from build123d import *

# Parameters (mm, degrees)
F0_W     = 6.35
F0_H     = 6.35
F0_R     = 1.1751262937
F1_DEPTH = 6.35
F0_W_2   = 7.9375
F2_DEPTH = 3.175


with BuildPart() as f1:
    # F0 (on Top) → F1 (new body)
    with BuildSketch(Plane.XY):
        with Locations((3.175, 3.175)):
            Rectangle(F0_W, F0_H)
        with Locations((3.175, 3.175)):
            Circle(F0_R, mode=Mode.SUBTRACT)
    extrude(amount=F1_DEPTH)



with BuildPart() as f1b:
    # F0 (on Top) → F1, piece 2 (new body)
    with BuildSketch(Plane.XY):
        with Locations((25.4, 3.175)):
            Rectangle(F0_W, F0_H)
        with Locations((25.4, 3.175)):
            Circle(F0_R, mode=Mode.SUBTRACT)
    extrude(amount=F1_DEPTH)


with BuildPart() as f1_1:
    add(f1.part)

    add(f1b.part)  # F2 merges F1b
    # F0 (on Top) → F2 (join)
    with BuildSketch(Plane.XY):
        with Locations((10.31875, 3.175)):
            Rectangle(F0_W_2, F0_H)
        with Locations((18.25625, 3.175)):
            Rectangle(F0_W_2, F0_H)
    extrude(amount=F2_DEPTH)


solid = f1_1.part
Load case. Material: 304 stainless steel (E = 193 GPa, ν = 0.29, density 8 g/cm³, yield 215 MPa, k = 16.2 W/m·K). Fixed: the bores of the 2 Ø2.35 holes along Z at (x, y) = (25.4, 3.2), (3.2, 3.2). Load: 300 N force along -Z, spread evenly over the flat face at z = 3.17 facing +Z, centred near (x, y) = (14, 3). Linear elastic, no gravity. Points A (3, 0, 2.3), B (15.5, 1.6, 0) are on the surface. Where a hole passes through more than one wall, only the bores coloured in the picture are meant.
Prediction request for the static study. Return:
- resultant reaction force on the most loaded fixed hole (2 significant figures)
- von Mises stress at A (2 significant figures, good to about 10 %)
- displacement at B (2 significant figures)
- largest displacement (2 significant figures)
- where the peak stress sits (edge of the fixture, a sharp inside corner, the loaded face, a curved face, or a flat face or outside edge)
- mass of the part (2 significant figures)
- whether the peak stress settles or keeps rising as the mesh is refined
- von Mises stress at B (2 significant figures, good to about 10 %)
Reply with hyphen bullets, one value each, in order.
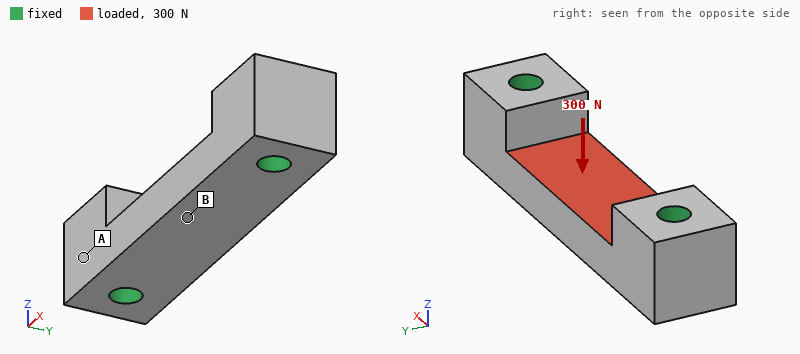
- 150 N
- 5.1 MPa
- 2.4 µm
- 2.5 µm
- edge of the fixture
- 6.2 g
- keeps rising
- 26 MPa
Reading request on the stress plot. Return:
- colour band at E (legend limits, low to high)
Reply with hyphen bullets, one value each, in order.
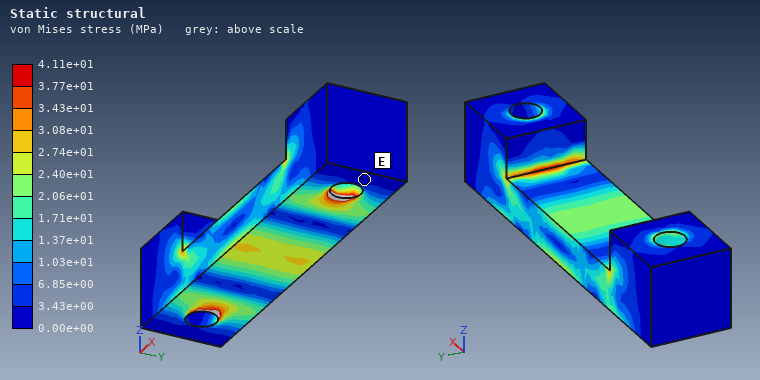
- 0.00e+00 to 3.43e+00 MPa
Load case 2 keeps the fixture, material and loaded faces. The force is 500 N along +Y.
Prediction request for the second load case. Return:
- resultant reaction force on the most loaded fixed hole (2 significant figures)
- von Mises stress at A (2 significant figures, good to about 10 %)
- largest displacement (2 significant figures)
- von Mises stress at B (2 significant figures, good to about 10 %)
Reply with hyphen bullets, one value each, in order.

- 250 N
- 14 MPa
- 4.1 µm
- 20 MPa
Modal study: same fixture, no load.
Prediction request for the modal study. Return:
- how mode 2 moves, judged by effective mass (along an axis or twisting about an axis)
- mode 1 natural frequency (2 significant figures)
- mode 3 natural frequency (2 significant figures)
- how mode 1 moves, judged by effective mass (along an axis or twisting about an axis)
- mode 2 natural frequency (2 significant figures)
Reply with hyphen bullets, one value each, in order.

- along Y
- 39 kHz
- 65 kHz
- along Z
- 45 kHz
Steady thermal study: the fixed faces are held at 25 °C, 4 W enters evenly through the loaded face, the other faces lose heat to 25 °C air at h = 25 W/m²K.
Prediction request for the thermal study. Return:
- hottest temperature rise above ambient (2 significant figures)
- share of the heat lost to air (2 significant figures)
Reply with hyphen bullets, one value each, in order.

- 38 K
- 4.0 %
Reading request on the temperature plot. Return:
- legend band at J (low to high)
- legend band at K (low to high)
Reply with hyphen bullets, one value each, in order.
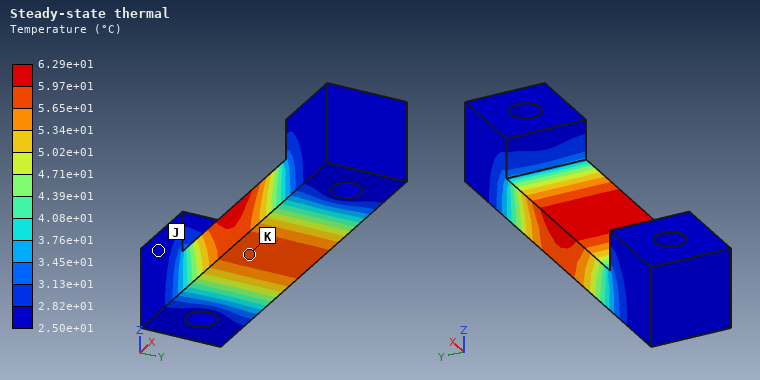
- 2.50e+01 to 2.82e+01 °C
- 5.65e+01 to 5.97e+01 °C
